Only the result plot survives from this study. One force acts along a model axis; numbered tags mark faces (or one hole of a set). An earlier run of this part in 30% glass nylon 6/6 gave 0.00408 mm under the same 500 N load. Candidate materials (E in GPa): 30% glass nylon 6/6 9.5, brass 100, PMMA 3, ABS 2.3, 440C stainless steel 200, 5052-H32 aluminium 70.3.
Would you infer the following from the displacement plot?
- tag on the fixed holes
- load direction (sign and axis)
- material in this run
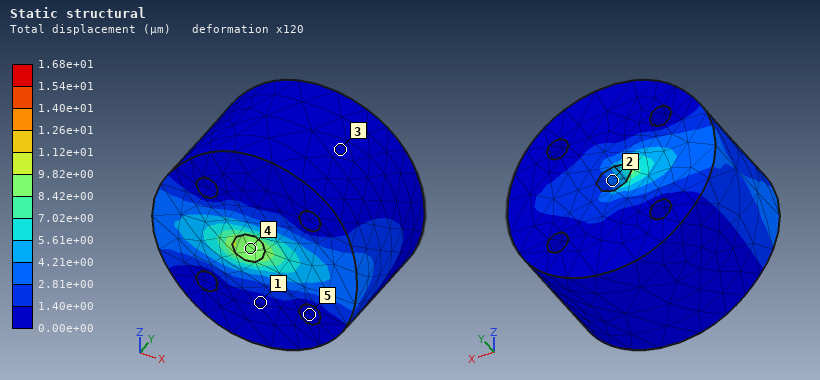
5
-X
ABS
